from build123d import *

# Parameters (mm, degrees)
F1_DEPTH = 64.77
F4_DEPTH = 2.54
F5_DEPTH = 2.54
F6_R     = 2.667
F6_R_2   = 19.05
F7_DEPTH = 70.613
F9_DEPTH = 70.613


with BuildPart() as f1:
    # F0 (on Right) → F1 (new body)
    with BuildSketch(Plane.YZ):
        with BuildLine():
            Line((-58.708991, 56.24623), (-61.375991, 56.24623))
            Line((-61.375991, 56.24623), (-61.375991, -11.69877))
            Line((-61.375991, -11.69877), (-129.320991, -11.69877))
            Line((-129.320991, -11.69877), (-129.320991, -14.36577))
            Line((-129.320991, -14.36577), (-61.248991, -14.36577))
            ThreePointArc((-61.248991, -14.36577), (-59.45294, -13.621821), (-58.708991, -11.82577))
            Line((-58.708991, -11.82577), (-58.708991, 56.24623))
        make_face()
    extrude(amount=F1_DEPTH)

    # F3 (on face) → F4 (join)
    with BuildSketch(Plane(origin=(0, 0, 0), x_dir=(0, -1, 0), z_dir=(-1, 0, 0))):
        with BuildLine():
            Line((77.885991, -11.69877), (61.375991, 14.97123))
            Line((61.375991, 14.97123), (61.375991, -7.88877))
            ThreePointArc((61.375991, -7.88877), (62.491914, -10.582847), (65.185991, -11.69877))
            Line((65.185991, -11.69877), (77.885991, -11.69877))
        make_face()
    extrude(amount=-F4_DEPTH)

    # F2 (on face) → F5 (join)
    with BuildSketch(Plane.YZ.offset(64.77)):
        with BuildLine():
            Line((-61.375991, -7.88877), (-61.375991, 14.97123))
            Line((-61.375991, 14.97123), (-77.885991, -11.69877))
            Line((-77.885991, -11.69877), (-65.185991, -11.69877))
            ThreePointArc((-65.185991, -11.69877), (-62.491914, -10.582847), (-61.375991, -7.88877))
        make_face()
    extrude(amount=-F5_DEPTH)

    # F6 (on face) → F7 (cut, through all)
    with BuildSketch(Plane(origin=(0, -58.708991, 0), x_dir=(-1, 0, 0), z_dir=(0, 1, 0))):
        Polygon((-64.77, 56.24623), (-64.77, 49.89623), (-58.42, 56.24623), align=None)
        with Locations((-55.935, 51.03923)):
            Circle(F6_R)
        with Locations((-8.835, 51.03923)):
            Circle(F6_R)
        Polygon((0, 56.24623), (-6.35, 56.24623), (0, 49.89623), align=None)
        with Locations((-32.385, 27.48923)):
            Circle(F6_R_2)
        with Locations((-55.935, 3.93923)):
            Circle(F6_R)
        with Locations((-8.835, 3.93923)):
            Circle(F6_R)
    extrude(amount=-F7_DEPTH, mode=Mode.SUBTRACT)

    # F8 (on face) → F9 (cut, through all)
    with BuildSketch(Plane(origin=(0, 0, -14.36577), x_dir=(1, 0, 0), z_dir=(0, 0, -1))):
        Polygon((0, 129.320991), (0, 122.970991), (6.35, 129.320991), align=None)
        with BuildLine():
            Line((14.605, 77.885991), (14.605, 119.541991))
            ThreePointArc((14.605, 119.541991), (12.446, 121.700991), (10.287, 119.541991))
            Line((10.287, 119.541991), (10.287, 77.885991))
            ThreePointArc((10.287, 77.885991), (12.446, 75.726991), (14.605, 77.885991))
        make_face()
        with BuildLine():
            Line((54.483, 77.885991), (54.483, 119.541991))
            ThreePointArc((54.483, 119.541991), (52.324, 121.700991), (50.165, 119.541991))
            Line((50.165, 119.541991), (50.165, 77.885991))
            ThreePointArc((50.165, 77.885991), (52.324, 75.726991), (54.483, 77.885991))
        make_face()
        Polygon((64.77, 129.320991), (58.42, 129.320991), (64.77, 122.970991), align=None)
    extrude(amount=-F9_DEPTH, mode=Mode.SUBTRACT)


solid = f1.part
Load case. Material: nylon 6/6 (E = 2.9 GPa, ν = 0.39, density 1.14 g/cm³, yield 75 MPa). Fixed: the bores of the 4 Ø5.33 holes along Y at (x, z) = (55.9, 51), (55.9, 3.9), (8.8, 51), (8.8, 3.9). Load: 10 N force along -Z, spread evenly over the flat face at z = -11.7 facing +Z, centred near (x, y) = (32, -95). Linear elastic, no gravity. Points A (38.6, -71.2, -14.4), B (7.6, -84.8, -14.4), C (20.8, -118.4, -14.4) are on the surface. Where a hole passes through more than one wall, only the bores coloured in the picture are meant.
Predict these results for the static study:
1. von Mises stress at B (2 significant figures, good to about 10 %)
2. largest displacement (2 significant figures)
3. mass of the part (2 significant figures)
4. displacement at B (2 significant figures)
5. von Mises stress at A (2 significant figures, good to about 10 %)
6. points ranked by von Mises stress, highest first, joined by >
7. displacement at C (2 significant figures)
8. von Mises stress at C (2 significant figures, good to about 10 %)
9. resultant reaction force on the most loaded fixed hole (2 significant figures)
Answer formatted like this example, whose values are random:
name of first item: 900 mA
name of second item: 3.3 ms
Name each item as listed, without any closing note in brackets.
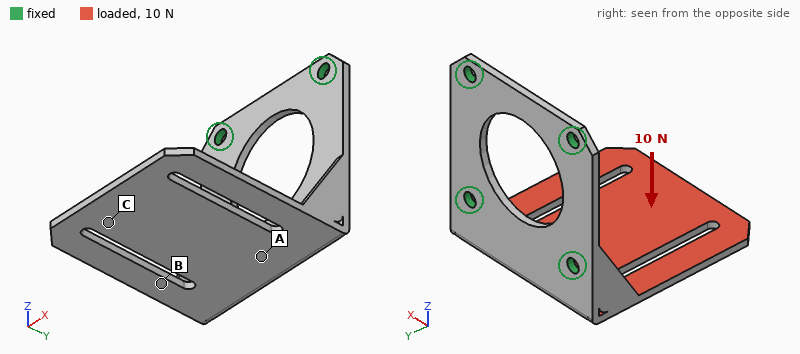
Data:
von Mises stress at B: 3.2 MPa
largest displacement: 1.3 mm
mass of the part: 23 g
displacement at B: 0.22 mm
von Mises stress at A: 1.8 MPa
points ranked by von Mises stress, highest first, joined by >: B > A > C
displacement at C: 1.1 mm
von Mises stress at C: 0.63 MPa
resultant reaction force on the most loaded fixed hole: 5.8 N
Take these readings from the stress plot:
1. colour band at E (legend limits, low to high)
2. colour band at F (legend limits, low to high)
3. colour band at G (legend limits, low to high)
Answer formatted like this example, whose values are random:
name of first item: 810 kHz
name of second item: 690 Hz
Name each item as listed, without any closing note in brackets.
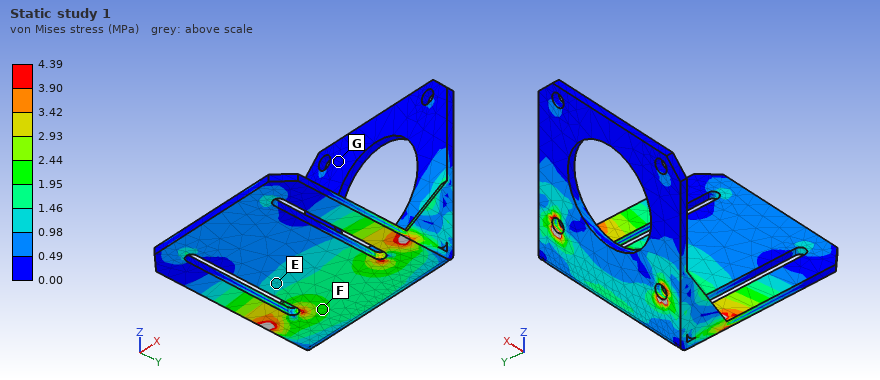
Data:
colour band at E: 0.98 to 1.46 MPa
colour band at F: 1.95 to 2.44 MPa
colour band at G: 0.00 to 0.49 MPa
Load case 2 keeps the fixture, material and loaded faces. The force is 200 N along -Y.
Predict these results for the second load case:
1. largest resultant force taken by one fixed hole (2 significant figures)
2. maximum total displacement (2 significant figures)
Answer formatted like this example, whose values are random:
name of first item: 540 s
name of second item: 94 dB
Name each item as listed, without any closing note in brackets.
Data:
largest resultant force taken by one fixed hole: 110 N
maximum total displacement: 1.2 mm
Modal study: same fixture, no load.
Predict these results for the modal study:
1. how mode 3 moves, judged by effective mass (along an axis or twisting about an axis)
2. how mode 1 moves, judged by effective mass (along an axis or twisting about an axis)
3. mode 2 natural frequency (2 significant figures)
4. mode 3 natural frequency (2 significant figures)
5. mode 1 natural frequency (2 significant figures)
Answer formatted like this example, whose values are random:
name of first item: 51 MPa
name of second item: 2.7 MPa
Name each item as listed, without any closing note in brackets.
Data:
how mode 3 moves, judged by effective mass: along X
how mode 1 moves, judged by effective mass: along Z
mode 2 natural frequency: 400 Hz
mode 3 natural frequency: 600 Hz
mode 1 natural frequency: 160 Hz
